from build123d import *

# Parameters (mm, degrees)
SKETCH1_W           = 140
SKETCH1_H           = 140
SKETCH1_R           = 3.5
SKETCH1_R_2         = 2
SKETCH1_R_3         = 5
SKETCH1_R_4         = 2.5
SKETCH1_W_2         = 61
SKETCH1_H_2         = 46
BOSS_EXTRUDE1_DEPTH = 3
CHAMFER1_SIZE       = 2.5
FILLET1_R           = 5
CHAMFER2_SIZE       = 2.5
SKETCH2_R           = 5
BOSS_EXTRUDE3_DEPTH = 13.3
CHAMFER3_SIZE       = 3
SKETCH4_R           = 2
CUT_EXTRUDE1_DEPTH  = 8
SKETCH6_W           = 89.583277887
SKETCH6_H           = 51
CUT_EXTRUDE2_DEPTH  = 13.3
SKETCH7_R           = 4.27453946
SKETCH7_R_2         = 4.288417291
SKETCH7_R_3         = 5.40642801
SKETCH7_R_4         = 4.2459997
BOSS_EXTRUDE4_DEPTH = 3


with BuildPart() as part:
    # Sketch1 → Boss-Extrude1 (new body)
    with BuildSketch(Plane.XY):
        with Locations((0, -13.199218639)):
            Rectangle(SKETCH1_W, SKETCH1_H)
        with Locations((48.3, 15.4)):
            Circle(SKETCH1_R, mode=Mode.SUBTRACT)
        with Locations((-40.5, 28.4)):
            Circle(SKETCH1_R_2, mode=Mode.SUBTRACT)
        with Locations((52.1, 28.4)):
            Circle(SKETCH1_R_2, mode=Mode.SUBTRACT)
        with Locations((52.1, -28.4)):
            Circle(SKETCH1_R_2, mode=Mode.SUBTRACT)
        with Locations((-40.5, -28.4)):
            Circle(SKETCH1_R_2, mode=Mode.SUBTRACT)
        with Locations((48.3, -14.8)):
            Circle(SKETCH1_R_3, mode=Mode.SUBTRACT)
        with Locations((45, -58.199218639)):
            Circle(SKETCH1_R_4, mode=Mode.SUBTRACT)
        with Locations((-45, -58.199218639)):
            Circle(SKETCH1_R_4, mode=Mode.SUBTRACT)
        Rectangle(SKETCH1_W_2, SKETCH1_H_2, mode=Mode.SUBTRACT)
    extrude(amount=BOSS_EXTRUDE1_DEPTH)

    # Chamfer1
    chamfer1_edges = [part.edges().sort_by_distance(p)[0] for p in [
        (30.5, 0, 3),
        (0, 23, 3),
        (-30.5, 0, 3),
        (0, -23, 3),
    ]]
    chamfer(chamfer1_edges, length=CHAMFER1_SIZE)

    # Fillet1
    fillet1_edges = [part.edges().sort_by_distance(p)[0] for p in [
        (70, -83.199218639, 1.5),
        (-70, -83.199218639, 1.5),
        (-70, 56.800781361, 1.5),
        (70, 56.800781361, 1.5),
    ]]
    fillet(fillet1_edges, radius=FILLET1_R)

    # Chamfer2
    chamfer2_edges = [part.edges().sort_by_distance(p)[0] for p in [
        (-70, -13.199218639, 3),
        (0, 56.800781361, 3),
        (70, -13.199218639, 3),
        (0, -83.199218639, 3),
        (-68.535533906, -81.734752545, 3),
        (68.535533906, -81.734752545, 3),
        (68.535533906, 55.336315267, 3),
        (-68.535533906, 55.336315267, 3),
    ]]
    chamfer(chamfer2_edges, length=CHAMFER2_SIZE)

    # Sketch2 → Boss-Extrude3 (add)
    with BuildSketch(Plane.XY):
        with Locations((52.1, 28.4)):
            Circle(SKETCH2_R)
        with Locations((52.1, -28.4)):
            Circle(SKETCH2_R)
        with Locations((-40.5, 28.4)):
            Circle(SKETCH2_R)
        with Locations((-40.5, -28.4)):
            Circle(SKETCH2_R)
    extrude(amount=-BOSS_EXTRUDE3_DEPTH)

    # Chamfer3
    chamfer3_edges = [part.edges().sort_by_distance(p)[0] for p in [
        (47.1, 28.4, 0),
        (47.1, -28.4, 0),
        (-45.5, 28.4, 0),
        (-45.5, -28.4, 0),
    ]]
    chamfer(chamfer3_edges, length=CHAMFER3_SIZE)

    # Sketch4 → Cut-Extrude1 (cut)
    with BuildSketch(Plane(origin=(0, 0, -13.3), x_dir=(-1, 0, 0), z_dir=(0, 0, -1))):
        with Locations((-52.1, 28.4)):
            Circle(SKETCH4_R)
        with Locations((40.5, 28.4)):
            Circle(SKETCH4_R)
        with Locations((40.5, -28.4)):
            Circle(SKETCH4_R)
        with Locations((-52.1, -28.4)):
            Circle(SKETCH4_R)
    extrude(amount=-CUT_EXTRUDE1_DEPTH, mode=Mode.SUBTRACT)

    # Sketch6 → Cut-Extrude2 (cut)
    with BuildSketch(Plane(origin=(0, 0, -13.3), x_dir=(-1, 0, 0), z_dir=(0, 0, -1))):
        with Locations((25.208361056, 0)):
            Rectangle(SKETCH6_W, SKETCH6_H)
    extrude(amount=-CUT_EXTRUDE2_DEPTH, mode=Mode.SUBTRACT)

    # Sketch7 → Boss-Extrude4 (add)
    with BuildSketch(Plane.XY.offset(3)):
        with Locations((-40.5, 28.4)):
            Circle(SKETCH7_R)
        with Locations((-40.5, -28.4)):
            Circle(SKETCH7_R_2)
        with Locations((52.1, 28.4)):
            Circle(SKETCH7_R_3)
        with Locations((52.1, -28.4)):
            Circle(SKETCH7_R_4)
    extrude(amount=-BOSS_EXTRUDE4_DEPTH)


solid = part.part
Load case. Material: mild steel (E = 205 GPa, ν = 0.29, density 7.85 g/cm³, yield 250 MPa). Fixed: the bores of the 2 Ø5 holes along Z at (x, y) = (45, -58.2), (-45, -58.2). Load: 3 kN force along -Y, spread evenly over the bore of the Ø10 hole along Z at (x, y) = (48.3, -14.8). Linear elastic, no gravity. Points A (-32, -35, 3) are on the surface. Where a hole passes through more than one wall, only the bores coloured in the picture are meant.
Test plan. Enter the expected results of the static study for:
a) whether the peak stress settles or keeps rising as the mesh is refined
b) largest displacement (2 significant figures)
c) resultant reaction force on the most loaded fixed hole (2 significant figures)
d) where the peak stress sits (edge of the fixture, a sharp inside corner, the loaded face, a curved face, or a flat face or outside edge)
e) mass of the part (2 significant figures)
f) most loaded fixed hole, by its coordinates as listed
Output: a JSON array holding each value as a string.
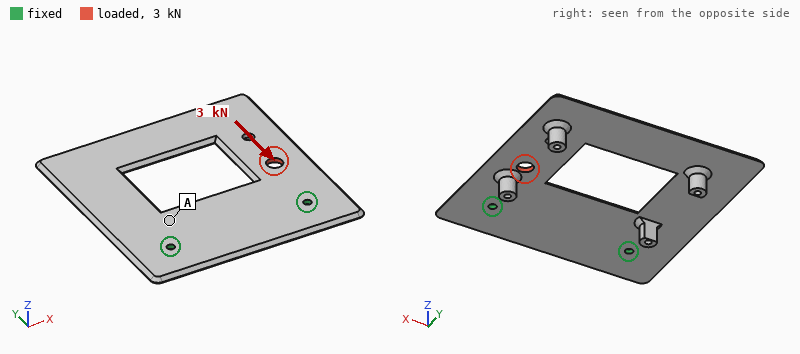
["keeps rising", "24 µm", "3.1 kN", "edge of the fixture", "400 g", "(45, -58.2)"]
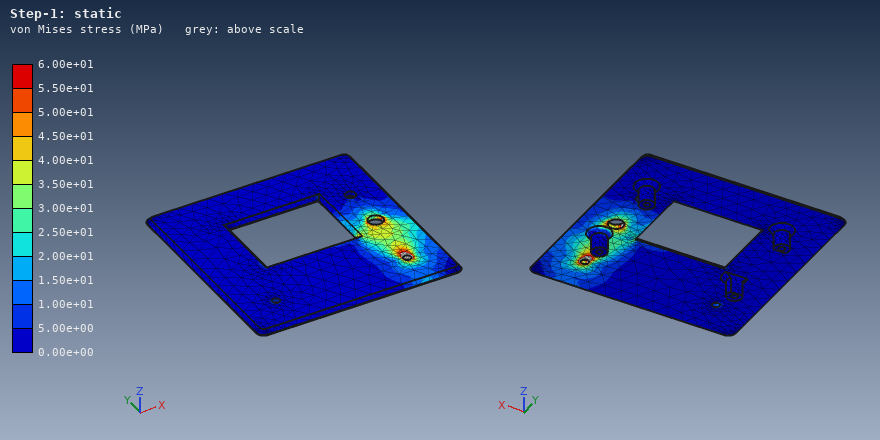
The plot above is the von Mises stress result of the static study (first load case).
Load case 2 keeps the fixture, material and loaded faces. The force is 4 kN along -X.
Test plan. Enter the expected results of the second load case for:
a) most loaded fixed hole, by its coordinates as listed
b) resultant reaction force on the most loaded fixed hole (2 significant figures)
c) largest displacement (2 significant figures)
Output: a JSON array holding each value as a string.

["(45, -58.2)", "3.0 kN", "37 µm"]
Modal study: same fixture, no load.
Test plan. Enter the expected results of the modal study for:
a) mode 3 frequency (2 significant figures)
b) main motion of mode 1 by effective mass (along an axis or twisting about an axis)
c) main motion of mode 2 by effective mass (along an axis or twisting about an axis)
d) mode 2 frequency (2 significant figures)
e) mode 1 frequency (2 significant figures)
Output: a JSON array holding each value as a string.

["910 Hz", "along Z", "twisting about Y", "350 Hz", "160 Hz"]
